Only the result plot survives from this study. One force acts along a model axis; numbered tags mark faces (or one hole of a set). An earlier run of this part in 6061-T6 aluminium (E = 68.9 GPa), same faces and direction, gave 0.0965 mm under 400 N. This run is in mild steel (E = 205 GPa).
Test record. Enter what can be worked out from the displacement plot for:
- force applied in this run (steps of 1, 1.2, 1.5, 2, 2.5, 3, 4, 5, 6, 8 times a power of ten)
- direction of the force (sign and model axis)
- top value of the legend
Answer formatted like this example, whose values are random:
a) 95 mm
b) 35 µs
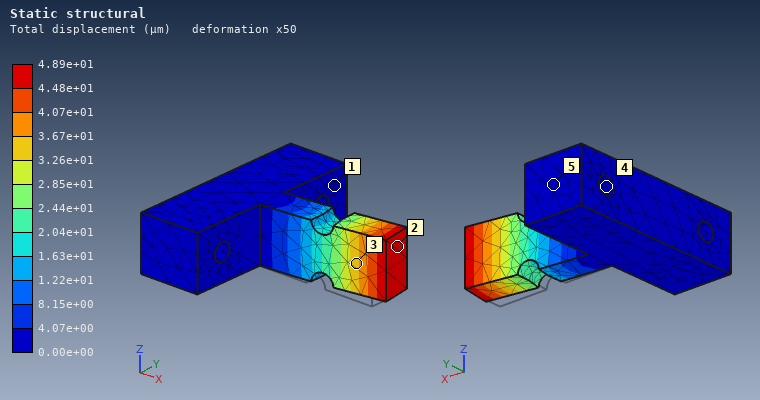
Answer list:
a) 600 N
b) +Y
c) 4.89e+01 µm
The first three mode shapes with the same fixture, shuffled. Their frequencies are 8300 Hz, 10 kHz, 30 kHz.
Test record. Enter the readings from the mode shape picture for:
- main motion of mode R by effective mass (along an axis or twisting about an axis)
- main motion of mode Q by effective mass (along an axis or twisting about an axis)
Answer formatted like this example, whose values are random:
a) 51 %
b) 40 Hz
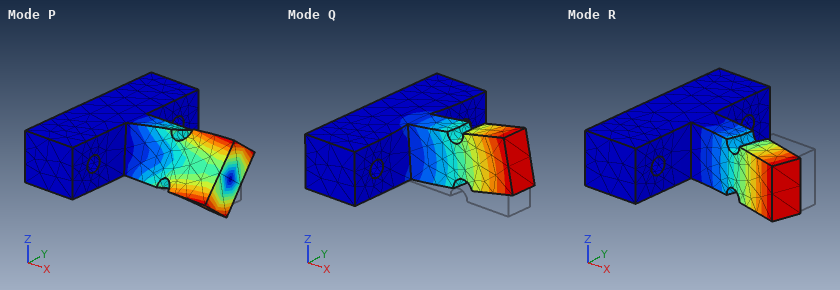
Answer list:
a) along Y
b) along Z
